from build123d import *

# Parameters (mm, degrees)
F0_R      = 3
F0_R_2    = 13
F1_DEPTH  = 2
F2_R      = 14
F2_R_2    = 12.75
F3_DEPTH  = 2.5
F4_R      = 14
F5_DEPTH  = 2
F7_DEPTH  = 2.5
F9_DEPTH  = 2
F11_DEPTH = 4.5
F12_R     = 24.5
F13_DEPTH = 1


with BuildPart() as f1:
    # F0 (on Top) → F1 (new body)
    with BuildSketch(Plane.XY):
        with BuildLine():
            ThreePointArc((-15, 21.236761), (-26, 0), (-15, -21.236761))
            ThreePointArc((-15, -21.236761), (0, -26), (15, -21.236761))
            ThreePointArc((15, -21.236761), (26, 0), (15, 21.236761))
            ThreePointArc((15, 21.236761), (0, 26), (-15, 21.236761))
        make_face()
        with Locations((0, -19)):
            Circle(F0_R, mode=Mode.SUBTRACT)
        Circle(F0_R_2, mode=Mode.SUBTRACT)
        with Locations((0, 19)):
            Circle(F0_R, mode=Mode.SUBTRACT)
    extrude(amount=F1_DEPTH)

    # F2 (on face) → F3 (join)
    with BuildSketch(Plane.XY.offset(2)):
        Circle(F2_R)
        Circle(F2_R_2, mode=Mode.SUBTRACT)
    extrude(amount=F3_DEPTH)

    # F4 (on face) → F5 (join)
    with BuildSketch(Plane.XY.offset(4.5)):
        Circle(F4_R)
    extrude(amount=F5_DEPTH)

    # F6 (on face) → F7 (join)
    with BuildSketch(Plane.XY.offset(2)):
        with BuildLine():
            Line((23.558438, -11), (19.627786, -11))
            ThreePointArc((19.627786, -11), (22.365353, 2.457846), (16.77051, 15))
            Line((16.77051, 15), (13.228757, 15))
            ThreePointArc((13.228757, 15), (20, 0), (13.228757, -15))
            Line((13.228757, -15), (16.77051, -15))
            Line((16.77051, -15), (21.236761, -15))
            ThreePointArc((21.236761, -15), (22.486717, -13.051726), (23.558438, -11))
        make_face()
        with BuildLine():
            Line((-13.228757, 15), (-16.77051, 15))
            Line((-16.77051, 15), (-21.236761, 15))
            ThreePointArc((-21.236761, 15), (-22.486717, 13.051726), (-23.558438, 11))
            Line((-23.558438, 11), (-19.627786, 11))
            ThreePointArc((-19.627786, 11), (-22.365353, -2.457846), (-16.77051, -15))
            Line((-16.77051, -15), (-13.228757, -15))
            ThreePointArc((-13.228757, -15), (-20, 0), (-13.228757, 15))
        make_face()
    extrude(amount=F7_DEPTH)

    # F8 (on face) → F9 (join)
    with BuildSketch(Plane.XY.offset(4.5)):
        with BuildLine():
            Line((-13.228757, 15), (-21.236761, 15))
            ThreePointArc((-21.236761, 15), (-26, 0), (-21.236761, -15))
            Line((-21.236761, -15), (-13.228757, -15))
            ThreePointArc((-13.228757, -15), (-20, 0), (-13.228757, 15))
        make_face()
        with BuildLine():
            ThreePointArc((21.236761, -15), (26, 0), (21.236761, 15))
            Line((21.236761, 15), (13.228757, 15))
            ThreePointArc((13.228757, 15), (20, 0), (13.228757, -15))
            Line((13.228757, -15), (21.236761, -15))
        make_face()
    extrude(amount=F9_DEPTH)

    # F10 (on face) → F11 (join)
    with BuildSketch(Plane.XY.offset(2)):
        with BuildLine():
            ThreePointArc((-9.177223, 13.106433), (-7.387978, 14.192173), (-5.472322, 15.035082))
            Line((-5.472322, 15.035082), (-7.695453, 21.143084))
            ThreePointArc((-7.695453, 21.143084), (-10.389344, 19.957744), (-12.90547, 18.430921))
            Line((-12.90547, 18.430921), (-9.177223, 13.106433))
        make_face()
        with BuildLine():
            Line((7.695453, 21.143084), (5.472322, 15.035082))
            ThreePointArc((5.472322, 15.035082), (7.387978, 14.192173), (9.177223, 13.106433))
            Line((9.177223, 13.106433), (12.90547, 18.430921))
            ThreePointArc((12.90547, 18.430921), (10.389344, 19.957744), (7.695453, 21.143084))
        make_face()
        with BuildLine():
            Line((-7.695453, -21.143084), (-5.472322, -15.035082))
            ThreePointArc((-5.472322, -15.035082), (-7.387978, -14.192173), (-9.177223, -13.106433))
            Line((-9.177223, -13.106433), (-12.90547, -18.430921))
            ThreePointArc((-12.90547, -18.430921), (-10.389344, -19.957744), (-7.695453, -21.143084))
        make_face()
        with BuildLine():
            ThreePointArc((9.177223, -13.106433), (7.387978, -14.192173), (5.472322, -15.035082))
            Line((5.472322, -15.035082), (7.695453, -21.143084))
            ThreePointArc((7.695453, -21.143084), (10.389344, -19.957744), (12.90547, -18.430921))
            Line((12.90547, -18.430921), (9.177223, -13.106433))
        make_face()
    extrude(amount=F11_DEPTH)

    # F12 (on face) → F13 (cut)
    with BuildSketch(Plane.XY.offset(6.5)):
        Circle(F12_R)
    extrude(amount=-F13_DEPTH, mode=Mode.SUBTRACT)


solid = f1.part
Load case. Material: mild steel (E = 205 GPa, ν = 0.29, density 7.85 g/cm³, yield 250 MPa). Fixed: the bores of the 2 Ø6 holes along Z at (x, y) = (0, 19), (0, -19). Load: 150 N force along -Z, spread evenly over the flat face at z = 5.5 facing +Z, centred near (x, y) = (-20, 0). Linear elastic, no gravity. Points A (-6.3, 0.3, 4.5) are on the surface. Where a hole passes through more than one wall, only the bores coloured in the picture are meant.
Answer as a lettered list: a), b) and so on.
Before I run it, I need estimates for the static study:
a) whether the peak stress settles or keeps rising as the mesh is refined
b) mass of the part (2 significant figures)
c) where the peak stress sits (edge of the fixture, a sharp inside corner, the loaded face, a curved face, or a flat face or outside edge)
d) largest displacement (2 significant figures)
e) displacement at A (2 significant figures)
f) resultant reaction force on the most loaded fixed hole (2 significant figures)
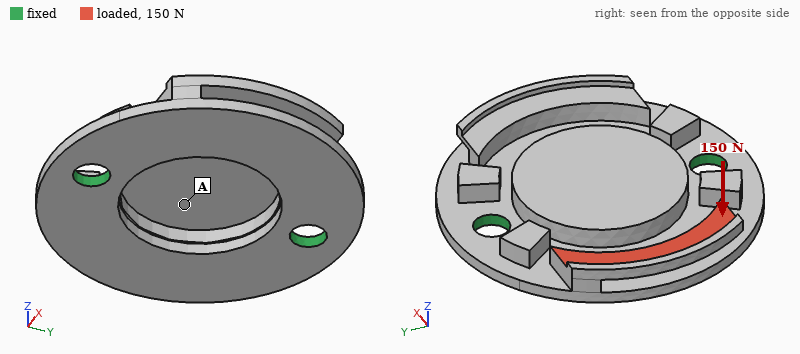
a) keeps rising
b) 42 g
c) edge of the fixture
d) 52 µm
e) 9.7 µm
f) 190 N
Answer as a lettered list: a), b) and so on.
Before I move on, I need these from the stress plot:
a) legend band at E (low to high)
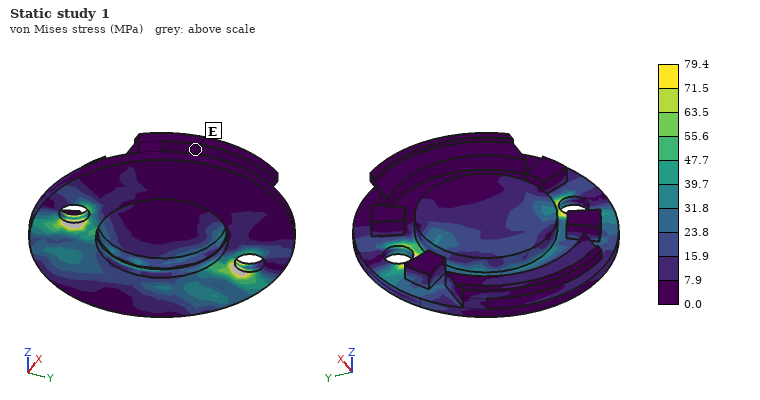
a) 0.0 to 7.9 MPa
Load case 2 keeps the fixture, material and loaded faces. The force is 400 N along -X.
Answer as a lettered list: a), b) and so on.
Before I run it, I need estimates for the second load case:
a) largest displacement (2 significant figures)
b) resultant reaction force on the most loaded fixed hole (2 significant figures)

a) 52 µm
b) 210 N
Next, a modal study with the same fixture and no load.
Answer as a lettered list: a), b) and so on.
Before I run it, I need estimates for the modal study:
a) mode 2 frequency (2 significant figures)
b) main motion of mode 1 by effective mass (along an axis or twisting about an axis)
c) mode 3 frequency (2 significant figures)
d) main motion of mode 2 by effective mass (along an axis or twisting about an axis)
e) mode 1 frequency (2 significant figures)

a) 4100 Hz
b) twisting about Y
c) 8100 Hz
d) along Z
e) 2800 Hz
